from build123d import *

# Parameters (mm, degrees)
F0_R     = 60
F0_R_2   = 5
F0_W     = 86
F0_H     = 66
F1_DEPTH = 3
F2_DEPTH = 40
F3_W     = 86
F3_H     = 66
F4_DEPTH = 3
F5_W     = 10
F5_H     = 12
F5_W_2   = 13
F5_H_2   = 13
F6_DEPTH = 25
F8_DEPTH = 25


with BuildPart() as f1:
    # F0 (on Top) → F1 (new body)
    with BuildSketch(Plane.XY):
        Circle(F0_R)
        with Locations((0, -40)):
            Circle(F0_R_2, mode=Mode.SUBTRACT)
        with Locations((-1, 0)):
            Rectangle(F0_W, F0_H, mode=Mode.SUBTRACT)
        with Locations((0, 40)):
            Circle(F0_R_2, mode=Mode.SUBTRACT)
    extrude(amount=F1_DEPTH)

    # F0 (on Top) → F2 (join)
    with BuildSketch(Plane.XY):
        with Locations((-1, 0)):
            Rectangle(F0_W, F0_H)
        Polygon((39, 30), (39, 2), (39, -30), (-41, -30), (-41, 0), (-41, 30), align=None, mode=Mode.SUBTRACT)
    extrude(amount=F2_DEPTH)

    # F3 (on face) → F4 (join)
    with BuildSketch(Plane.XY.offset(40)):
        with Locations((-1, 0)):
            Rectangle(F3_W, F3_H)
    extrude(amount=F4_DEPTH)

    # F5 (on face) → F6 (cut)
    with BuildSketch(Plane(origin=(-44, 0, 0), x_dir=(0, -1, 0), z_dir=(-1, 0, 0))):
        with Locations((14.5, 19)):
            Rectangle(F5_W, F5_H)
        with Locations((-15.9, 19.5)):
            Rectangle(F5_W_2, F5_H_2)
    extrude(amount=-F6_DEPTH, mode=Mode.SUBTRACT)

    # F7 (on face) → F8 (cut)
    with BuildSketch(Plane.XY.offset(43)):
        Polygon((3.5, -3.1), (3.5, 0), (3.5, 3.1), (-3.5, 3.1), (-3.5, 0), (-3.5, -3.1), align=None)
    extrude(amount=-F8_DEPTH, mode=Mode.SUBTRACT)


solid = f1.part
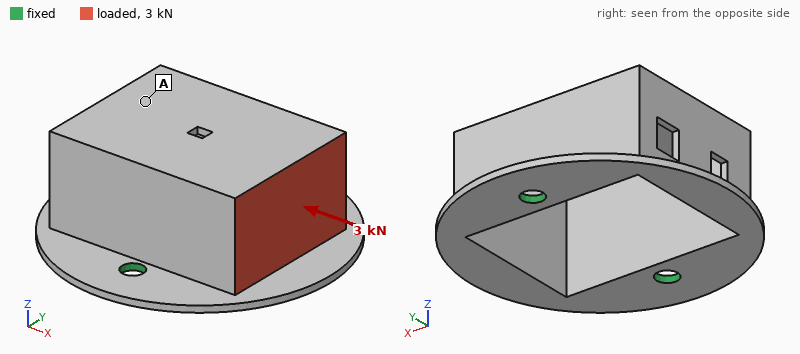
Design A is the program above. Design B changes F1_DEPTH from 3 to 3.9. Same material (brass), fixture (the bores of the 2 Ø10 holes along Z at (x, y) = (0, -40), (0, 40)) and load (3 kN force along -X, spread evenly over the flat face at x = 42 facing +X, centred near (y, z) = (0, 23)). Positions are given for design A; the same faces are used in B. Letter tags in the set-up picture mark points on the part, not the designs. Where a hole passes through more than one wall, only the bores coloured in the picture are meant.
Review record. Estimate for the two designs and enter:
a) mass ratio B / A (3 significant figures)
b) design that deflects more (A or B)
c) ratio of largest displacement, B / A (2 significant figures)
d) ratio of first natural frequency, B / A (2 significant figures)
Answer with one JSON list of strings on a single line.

["1.07", "A", "0.63", "1.3"]
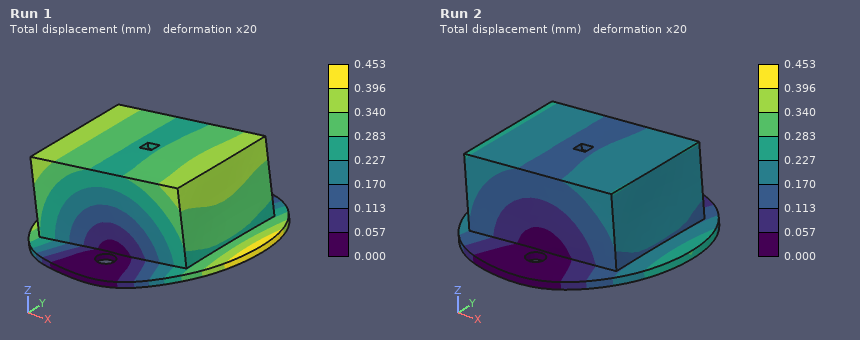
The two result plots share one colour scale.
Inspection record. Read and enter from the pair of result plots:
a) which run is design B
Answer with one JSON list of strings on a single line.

["Run 2"]
